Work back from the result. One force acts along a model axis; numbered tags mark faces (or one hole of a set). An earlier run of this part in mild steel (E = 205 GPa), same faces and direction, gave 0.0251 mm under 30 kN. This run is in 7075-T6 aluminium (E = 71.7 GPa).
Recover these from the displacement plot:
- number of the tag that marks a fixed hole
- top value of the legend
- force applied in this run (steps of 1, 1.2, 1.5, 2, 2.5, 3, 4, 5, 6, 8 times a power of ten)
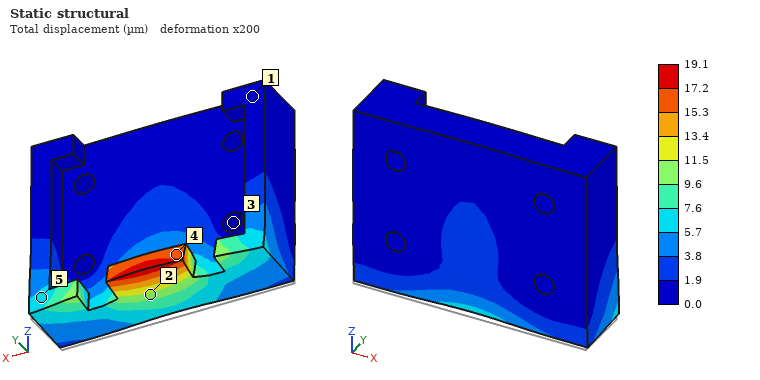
3
19.1 µm
8 kN
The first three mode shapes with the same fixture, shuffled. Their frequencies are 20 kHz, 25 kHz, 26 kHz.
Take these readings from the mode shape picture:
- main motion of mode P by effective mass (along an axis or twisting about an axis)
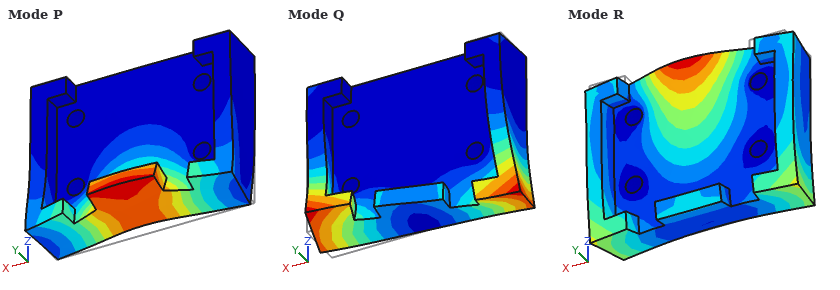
along Y
